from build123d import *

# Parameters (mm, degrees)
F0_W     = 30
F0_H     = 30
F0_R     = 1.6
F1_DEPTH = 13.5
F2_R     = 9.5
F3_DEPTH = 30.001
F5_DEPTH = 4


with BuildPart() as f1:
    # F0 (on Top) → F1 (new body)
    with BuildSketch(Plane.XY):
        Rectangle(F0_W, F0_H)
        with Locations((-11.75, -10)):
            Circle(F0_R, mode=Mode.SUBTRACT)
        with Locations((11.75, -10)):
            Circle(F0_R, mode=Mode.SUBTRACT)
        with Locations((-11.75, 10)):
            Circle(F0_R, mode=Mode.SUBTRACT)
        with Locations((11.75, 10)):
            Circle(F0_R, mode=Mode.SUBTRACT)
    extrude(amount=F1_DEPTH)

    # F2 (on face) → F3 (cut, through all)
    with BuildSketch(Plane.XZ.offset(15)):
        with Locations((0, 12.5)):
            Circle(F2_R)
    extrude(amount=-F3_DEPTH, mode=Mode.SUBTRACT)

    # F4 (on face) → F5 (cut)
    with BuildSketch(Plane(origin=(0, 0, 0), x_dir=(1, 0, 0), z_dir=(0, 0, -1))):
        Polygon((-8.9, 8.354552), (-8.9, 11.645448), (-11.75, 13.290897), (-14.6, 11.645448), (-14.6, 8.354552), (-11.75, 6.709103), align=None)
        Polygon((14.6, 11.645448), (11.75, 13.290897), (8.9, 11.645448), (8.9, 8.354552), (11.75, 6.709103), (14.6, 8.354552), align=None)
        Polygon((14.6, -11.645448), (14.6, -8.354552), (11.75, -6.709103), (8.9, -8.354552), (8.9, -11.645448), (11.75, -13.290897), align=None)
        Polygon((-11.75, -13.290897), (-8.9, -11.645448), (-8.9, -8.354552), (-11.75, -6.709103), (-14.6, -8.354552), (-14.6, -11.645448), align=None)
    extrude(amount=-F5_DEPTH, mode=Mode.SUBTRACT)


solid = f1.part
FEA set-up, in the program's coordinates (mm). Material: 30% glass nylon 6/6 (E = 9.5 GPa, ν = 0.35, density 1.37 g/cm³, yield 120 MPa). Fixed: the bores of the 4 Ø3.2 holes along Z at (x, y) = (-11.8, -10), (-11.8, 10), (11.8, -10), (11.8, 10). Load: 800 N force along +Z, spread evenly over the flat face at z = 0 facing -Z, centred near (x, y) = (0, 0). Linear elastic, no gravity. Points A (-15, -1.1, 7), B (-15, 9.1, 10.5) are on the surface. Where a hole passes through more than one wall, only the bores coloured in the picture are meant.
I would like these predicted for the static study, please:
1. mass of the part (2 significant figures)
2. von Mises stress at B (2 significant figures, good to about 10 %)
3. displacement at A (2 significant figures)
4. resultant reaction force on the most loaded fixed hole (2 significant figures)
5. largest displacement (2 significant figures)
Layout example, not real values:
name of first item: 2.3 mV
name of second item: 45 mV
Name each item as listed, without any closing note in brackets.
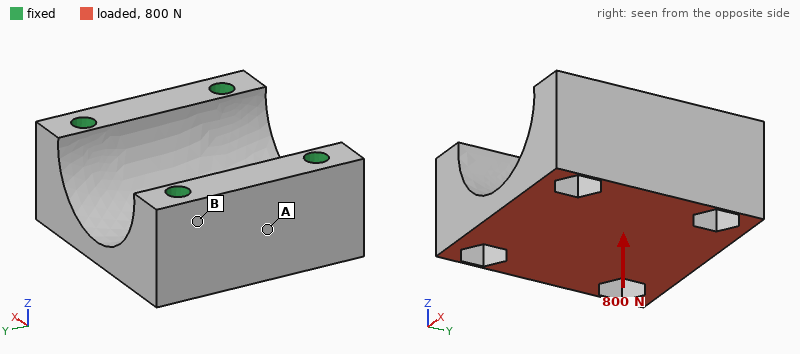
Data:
mass of the part: 9.0 g
von Mises stress at B: 1.9 MPa
displacement at A: 2.3 µm
resultant reaction force on the most loaded fixed hole: 230 N
largest displacement: 10 µm
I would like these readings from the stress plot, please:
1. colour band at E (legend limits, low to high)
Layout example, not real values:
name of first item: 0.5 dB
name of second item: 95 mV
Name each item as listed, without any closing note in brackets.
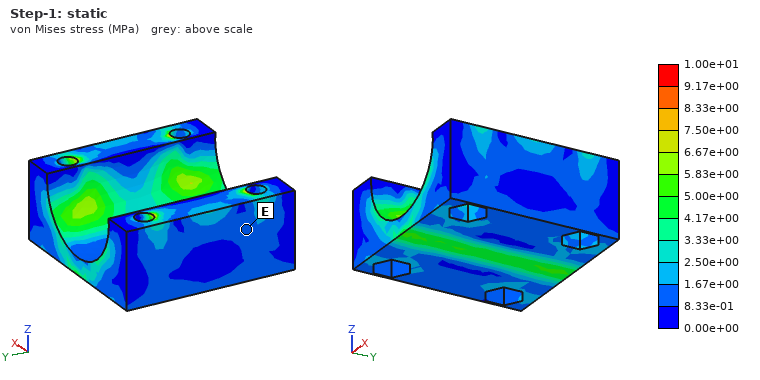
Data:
colour band at E: 8.33e-01 to 1.67e+00 MPa
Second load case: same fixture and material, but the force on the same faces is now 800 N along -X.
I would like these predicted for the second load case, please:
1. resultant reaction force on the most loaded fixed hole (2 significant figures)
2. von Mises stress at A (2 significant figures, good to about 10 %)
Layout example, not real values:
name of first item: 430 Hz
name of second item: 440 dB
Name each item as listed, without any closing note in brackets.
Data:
resultant reaction force on the most loaded fixed hole: 220 N
von Mises stress at A: 2.0 MPa
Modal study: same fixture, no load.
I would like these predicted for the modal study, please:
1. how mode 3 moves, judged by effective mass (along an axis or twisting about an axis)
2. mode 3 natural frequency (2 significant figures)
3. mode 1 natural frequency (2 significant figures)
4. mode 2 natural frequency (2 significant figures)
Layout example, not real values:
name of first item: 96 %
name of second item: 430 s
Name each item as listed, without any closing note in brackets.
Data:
how mode 3 moves, judged by effective mass: along Y
mode 3 natural frequency: 27 kHz
mode 1 natural frequency: 24 kHz
mode 2 natural frequency: 25 kHz
